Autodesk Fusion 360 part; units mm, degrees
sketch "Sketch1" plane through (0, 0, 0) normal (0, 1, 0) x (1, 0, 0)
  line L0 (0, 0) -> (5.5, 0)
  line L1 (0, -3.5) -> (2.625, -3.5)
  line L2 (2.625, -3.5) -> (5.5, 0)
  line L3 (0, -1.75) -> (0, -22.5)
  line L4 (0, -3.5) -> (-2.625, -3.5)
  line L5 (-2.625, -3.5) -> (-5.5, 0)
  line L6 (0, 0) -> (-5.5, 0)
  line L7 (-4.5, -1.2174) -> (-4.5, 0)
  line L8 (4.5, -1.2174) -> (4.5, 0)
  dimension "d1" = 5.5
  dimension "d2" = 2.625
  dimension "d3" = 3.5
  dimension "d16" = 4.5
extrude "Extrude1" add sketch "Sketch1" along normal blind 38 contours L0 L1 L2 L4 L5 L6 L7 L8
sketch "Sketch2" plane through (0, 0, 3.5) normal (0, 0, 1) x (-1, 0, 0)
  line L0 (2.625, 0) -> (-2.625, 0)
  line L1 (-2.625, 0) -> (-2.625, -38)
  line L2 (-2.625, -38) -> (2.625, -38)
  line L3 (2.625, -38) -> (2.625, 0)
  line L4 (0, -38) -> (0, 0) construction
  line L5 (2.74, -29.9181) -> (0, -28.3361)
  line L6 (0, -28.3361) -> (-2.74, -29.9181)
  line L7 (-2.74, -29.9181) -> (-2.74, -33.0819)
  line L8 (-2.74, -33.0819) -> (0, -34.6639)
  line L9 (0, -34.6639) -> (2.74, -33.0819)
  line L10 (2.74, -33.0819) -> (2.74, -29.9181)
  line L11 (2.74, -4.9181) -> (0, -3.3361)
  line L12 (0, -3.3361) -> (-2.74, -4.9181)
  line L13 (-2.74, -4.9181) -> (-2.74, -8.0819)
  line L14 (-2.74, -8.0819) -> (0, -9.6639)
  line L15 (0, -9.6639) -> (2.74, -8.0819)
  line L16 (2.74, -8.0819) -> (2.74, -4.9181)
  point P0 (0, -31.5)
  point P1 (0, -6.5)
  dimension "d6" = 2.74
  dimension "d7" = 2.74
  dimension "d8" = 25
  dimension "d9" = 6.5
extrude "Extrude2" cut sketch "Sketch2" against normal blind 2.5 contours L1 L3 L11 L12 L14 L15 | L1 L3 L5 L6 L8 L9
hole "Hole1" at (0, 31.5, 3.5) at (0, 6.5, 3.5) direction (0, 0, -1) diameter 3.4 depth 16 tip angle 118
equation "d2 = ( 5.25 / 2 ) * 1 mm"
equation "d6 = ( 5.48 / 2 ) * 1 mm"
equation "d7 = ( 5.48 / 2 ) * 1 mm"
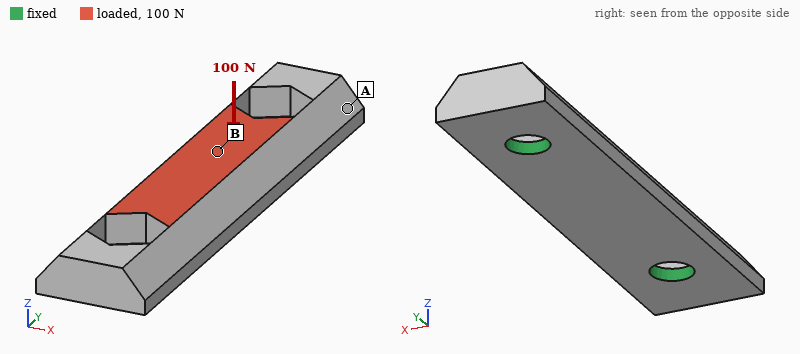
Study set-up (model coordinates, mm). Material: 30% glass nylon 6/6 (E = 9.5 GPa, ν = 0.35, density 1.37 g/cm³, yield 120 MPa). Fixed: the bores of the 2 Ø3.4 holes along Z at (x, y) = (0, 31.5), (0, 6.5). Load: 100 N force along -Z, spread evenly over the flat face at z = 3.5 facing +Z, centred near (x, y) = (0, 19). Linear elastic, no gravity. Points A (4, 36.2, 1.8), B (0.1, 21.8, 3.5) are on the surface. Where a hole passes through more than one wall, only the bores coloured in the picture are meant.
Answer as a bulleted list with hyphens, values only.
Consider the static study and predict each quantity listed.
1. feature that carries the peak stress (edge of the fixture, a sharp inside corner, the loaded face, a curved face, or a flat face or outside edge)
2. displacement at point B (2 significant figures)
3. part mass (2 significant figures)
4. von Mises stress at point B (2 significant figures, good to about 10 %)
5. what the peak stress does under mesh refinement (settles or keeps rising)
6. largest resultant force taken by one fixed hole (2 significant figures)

- edge of the fixture
- 34 µm
- 1.2 g
- 12 MPa
- keeps rising
- 78 N
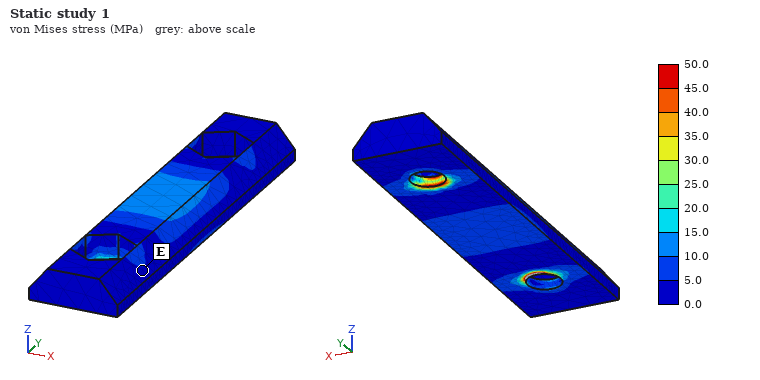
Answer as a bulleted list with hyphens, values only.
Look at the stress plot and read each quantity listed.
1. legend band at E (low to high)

- 0.0 to 5.0 MPa
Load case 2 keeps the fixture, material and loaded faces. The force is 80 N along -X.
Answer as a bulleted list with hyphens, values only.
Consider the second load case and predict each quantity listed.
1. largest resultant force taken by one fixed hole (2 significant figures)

- 40 N
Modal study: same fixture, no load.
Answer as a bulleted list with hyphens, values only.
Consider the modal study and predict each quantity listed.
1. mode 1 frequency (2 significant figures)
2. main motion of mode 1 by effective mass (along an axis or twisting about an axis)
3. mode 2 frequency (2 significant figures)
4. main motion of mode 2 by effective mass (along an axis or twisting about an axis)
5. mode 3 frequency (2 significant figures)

- 10 kHz
- along Z
- 13 kHz
- along X
- 16 kHz
